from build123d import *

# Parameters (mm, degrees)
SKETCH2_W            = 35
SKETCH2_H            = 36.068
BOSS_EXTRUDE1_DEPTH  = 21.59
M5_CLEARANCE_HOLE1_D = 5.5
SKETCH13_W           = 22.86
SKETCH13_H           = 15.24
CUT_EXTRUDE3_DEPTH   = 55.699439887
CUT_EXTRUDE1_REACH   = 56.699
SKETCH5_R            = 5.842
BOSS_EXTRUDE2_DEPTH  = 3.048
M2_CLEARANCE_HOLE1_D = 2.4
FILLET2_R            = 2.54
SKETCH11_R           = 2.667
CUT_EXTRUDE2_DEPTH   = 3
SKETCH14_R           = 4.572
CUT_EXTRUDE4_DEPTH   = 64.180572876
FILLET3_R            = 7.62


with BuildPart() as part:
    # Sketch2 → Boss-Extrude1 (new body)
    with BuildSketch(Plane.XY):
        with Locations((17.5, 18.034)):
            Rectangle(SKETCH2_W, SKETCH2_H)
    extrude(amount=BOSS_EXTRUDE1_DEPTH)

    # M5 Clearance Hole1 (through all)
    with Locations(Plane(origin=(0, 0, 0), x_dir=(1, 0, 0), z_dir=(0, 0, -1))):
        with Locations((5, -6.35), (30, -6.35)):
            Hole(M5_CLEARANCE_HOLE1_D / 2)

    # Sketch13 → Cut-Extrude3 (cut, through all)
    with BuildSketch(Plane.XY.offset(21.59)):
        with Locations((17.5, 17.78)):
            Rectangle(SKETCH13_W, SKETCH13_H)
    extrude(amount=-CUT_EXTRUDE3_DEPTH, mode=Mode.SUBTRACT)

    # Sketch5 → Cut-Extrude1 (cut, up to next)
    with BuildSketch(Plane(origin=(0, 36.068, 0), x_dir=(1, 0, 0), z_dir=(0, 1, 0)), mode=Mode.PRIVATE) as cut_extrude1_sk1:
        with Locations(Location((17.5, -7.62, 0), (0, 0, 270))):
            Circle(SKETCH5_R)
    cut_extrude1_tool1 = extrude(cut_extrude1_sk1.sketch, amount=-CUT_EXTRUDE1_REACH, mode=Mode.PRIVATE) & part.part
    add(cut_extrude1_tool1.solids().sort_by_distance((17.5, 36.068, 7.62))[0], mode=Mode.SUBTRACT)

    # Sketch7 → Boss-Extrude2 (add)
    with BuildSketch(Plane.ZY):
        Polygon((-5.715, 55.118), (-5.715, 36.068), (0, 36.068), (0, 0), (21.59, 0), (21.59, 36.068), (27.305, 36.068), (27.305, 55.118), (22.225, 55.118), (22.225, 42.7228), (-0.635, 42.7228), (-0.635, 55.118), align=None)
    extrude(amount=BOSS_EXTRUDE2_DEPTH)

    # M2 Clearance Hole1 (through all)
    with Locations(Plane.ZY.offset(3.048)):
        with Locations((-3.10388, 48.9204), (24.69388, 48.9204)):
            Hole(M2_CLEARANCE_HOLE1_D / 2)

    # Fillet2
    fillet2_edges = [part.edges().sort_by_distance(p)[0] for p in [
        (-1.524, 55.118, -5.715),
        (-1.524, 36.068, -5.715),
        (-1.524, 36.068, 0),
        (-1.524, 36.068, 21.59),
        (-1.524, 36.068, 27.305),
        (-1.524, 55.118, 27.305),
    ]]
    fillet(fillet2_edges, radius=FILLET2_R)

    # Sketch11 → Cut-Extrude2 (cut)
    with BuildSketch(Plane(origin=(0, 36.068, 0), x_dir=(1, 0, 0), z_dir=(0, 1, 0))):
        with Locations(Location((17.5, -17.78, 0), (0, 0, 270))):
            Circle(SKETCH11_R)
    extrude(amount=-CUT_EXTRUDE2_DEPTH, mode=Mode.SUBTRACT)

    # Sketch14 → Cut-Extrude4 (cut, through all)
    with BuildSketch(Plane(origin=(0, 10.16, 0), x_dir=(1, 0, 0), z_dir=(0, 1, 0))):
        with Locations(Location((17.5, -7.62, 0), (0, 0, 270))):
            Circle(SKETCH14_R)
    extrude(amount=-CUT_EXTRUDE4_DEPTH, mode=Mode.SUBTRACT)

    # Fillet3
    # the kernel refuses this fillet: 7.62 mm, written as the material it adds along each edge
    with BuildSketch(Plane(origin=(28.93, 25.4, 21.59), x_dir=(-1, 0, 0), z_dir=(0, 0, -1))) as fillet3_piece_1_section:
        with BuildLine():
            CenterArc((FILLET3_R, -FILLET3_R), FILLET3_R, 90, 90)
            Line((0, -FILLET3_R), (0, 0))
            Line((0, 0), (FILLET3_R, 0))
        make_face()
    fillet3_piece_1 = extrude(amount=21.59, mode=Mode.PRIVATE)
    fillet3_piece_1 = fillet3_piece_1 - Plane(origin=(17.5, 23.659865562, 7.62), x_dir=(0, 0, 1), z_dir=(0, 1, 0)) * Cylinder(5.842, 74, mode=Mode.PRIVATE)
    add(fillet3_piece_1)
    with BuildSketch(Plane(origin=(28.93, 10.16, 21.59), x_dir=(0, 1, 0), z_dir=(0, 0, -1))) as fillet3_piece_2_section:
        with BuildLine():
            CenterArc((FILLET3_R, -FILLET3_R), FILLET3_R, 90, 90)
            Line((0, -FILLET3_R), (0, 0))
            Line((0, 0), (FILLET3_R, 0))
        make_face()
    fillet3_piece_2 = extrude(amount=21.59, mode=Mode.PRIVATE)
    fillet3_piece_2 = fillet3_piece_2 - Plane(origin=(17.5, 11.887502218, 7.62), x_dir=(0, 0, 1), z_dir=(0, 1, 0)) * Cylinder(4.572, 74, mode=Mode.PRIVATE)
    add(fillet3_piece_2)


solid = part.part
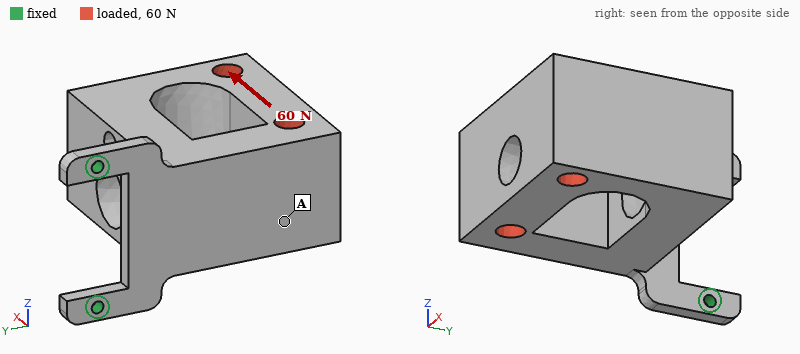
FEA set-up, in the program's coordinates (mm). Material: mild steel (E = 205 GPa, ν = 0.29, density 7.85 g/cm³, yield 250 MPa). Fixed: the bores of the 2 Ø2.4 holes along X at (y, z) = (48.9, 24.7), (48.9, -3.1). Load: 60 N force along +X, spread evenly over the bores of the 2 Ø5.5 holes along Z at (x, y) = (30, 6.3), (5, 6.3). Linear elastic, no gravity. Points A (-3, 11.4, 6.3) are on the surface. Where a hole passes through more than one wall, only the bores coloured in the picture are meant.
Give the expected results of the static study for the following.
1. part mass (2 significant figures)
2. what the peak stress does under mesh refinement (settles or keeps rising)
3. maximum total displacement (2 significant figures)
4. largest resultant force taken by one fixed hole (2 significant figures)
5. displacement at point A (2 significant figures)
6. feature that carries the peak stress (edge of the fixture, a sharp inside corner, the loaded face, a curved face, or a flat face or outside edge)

160 g
keeps rising
0.29 mm
30 N
0.16 mm
edge of the fixture
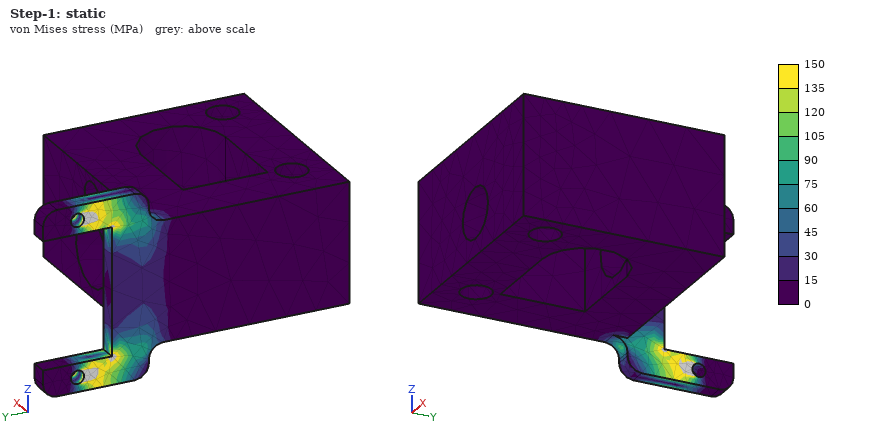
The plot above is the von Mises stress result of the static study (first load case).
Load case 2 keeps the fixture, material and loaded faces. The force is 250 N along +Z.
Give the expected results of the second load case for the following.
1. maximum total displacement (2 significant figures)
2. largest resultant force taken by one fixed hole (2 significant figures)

61 µm
410 N
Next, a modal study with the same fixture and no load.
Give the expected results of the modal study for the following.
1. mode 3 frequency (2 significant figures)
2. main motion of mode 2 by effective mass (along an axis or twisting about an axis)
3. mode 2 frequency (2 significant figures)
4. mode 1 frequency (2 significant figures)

2500 Hz
along Z
1000 Hz
240 Hz
